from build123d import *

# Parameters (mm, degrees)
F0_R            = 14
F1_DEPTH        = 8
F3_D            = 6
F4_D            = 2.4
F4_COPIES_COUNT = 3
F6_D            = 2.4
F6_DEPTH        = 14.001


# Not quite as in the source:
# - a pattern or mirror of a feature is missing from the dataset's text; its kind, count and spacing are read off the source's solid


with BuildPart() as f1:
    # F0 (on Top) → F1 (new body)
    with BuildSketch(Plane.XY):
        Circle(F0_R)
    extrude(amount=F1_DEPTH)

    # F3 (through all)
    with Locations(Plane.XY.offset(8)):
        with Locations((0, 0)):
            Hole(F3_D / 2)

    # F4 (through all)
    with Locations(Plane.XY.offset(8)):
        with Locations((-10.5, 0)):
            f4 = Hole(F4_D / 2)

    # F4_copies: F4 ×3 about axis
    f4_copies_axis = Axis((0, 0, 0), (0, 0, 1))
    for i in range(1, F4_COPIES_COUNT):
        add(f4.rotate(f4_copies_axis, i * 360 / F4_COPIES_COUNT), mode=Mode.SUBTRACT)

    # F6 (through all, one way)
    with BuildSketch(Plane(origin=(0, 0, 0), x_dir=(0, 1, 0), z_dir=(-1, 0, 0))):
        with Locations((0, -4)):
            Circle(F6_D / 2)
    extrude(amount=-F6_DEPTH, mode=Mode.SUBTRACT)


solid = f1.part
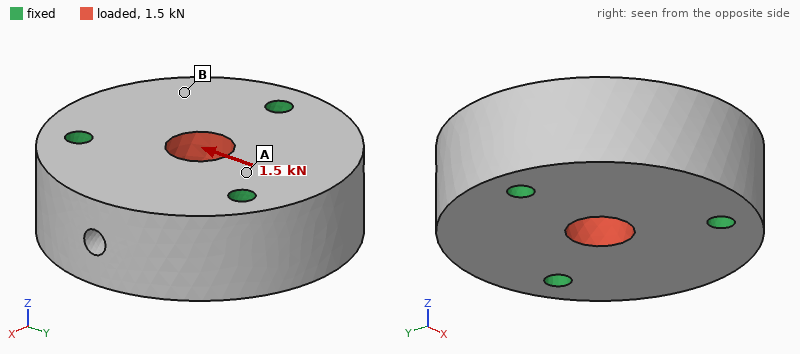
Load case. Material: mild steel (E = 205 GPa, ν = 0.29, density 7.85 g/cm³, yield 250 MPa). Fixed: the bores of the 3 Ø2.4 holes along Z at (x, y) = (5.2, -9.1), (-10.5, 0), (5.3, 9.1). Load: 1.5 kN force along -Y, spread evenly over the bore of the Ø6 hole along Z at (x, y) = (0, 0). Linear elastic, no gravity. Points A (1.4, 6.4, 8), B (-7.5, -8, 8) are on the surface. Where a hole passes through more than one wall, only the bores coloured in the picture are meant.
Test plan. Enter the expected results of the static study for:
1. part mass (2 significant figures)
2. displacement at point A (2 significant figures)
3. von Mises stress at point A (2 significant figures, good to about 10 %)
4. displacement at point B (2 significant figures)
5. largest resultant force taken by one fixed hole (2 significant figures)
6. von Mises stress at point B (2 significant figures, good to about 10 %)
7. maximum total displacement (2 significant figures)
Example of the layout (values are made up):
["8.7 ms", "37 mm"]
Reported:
["36 g", "0.30 µm", "9.5 MPa", "0.30 µm", "500 N", "4.4 MPa", "0.58 µm"]
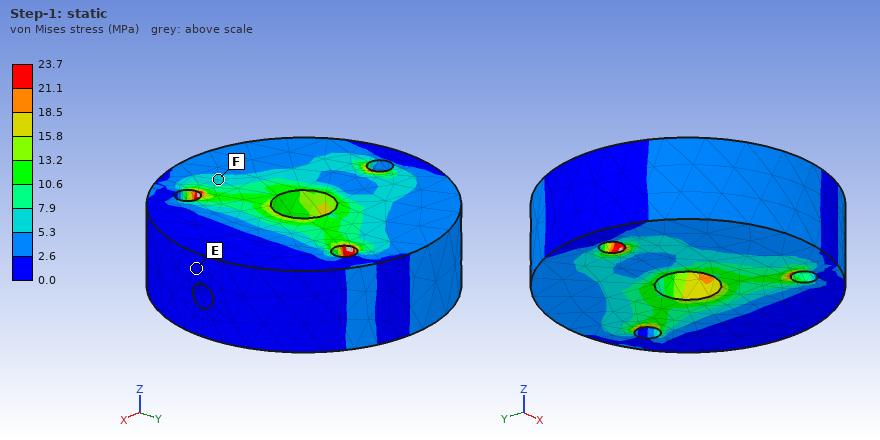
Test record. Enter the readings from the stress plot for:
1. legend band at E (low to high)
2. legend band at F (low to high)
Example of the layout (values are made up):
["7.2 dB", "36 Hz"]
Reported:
["0.0 to 2.6 MPa", "5.3 to 7.9 MPa"]
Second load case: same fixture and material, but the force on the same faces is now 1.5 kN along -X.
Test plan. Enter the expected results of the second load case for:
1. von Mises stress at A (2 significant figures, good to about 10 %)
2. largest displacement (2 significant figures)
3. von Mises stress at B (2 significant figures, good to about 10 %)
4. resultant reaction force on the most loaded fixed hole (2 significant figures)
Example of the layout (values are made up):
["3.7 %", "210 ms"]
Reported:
["5.3 MPa", "0.61 µm", "2.1 MPa", "530 N"]
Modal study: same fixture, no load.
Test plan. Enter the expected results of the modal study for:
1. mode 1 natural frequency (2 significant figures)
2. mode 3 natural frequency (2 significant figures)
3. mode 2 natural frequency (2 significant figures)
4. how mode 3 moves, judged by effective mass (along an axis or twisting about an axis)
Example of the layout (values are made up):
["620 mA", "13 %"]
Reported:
["47 kHz", "53 kHz", "48 kHz", "along Z"]
